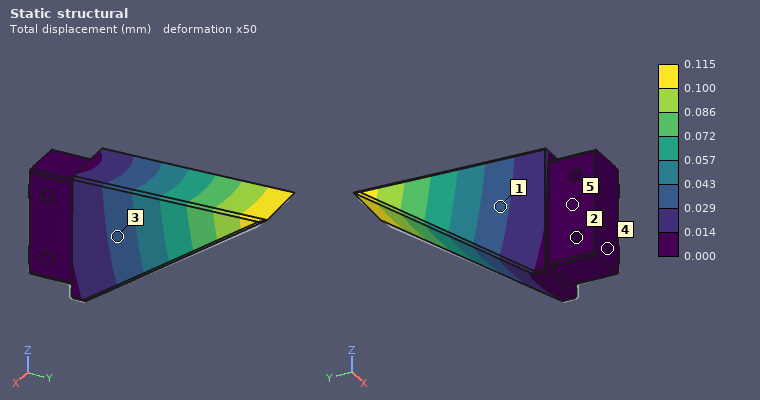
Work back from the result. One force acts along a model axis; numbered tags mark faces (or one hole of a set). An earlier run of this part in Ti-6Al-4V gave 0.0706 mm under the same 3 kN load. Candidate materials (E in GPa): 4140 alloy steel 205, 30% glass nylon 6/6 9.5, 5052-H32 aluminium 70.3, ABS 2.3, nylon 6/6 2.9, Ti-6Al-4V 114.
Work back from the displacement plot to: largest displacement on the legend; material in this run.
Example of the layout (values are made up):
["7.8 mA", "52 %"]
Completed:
["0.115 mm", "5052-H32 aluminium"]
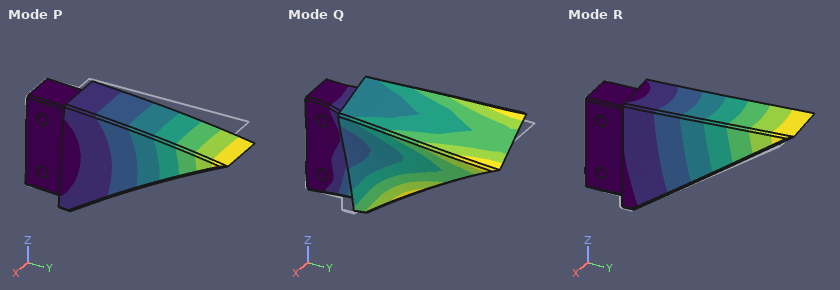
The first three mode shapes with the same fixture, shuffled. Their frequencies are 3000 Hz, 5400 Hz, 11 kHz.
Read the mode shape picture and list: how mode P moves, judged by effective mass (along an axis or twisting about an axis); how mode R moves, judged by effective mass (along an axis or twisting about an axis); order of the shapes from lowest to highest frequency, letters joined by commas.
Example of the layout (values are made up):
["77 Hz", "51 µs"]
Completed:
["along Z", "along X", "R, P, Q"]
